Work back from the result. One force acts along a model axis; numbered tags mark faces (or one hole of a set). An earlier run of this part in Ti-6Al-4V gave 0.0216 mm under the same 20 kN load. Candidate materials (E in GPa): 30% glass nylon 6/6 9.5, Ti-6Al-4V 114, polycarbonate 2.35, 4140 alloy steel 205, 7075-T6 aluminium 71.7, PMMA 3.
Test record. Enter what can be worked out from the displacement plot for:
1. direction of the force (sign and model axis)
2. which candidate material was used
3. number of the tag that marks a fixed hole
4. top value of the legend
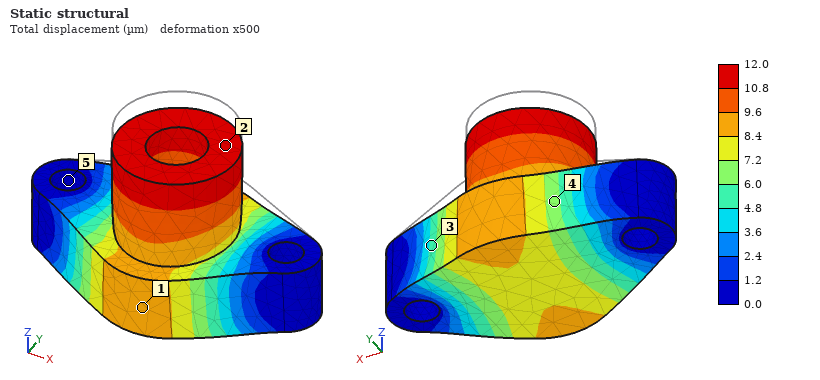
-Z
4140 alloy steel
5
12.0 µm
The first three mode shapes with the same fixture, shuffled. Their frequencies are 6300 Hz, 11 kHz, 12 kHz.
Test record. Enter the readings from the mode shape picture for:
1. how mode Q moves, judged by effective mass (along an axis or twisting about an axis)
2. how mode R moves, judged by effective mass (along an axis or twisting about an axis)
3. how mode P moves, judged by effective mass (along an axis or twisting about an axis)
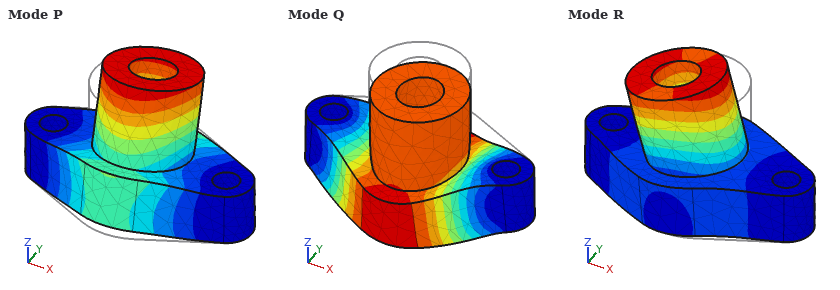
along Z
along X
along Y
